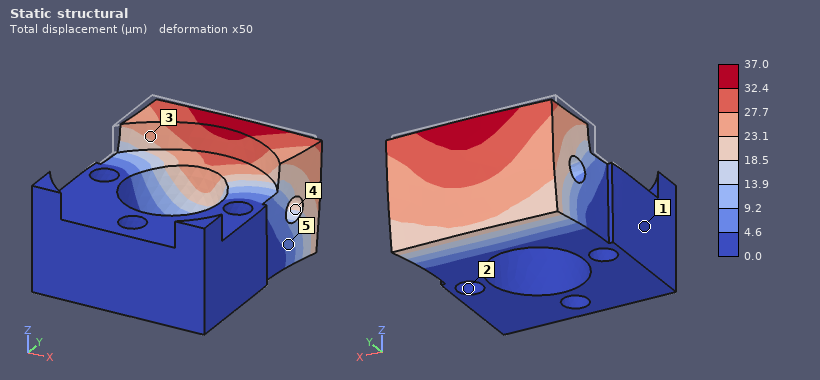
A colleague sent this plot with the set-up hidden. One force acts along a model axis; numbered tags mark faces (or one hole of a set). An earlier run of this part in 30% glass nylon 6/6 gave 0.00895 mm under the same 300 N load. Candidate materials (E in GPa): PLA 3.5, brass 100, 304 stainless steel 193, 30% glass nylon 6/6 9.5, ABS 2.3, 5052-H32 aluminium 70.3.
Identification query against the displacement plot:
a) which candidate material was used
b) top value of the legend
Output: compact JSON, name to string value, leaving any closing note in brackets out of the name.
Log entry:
{"which candidate material was used": "ABS", "top value of the legend": "37.0 µm"}
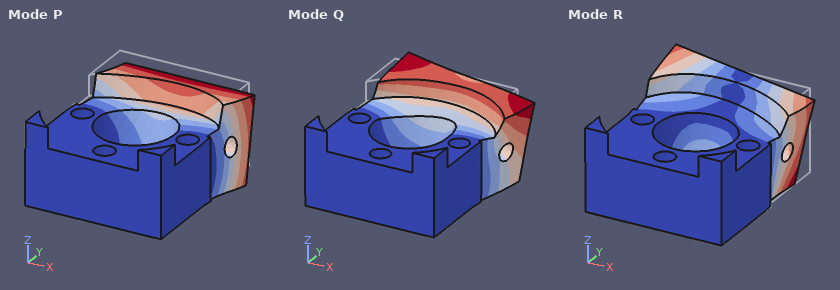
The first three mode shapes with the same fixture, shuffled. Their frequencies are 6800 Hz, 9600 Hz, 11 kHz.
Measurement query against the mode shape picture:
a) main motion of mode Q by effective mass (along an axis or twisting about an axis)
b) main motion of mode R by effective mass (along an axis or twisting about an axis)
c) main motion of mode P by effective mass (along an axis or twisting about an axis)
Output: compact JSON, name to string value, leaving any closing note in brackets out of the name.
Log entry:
{"main motion of mode Q by effective mass": "along X", "main motion of mode R by effective mass": "along X", "main motion of mode P by effective mass": "along Z"}
